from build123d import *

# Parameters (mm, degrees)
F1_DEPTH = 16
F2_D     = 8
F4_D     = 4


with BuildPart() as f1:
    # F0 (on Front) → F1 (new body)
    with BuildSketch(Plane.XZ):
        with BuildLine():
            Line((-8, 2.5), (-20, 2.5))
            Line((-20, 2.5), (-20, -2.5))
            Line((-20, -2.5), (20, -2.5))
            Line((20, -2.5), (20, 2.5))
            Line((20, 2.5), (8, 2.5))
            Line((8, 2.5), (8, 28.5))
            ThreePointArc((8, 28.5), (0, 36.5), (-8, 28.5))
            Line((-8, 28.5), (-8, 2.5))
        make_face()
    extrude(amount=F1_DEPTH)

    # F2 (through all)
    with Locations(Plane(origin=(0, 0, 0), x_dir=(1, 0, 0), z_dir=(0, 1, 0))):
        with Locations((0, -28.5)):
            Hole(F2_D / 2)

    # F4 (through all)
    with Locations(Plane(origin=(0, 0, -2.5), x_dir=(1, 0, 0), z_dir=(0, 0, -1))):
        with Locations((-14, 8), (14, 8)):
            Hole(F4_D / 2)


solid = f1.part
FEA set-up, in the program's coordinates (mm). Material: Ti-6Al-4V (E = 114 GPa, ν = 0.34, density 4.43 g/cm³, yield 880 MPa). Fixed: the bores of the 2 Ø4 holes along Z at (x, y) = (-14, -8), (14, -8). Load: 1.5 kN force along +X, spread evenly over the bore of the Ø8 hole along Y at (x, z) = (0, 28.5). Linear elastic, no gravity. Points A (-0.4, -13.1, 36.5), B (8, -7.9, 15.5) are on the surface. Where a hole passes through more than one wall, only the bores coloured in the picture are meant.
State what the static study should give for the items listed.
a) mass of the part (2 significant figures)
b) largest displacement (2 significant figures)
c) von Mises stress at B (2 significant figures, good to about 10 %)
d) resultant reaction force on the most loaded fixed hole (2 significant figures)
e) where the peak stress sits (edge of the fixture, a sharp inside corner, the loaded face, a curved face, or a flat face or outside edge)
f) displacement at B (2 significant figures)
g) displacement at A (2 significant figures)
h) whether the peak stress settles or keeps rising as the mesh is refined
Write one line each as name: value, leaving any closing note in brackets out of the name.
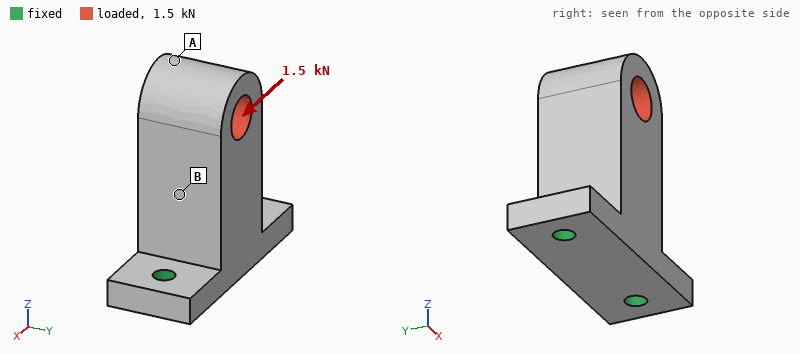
mass of the part: 47 g
largest displacement: 62 µm
von Mises stress at B: 30 MPa
resultant reaction force on the most loaded fixed hole: 2.1 kN
where the peak stress sits: edge of the fixture
displacement at B: 24 µm
displacement at A: 62 µm
whether the peak stress settles or keeps rising as the mesh is refined: keeps rising
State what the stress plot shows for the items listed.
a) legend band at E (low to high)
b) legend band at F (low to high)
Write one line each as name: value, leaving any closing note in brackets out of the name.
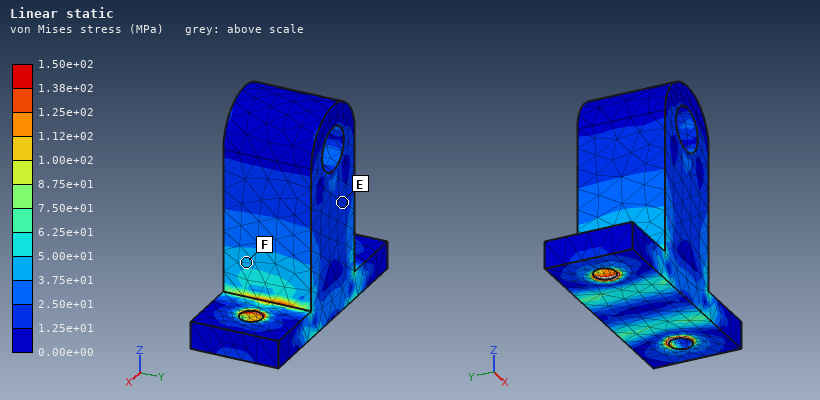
legend band at E: 1.25e+01 to 2.50e+01 MPa
legend band at F: 3.75e+01 to 5.00e+01 MPa
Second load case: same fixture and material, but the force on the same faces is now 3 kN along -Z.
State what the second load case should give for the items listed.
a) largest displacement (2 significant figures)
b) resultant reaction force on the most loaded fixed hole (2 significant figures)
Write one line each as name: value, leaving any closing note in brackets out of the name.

largest displacement: 13 µm
resultant reaction force on the most loaded fixed hole: 1.6 kN
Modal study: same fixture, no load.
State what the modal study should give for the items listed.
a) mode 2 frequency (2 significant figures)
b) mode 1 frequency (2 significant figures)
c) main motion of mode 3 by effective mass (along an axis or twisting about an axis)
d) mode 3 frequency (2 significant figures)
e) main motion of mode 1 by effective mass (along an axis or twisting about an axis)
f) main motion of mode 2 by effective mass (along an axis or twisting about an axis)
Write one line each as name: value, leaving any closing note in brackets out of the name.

mode 2 frequency: 7200 Hz
mode 1 frequency: 3600 Hz
main motion of mode 3 by effective mass: along Z
mode 3 frequency: 15 kHz
main motion of mode 1 by effective mass: along Y
main motion of mode 2 by effective mass: along X
